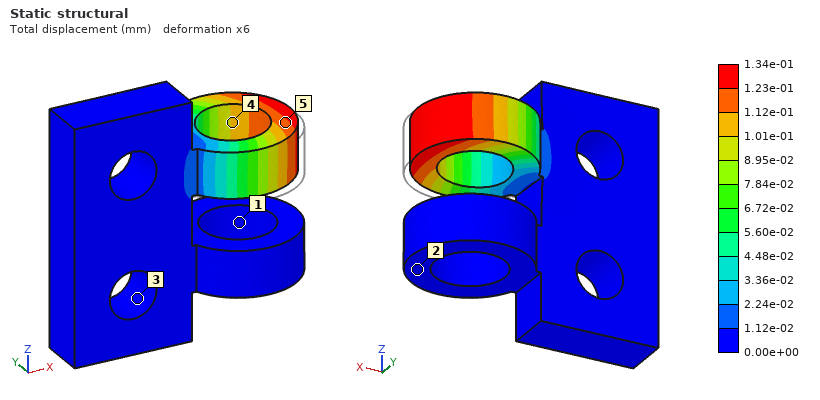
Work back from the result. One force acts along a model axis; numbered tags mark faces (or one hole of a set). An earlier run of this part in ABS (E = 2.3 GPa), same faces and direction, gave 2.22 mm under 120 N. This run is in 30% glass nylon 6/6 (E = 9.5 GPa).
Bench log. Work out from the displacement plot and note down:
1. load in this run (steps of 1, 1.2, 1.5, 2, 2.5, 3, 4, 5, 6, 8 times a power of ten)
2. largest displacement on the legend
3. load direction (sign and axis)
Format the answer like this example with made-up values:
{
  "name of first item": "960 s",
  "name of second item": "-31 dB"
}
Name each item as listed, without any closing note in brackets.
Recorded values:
{
  "load in this run": "30 N",
  "largest displacement on the legend": "1.34e-01 mm",
  "load direction": "+Y"
}
